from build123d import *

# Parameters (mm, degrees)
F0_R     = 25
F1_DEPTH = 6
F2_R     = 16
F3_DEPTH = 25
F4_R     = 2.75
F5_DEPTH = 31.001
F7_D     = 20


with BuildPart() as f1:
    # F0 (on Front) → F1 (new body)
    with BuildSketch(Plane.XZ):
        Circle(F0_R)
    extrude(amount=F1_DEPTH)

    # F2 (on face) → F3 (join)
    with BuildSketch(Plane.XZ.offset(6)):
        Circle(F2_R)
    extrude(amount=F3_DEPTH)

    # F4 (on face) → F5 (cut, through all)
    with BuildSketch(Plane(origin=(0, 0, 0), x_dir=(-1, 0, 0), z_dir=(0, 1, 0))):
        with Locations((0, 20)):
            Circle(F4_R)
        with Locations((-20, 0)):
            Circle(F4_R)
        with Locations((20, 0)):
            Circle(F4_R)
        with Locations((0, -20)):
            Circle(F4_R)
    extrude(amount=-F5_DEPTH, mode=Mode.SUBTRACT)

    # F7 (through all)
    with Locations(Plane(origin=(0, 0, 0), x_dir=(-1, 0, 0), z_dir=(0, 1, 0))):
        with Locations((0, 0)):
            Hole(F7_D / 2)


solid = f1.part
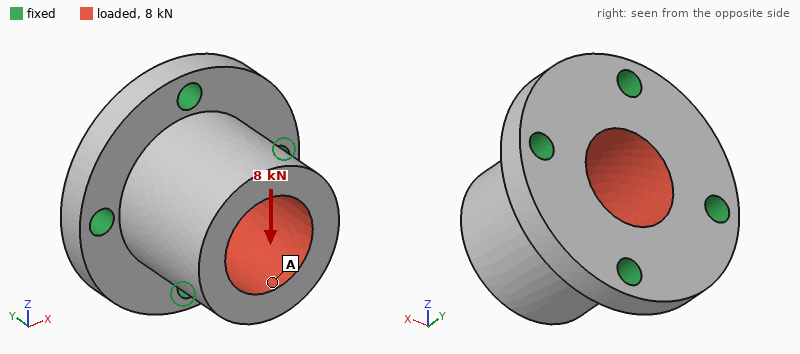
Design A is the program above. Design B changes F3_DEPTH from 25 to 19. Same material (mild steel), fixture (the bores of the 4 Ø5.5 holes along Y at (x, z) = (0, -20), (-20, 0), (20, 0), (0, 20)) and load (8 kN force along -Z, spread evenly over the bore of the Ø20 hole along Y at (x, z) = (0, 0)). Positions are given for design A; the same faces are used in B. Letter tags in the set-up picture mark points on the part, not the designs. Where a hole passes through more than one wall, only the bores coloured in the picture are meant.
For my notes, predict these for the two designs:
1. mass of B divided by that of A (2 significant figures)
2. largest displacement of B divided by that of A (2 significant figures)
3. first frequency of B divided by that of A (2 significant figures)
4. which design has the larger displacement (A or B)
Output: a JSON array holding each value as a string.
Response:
["0.86", "0.67", "1.3", "A"]
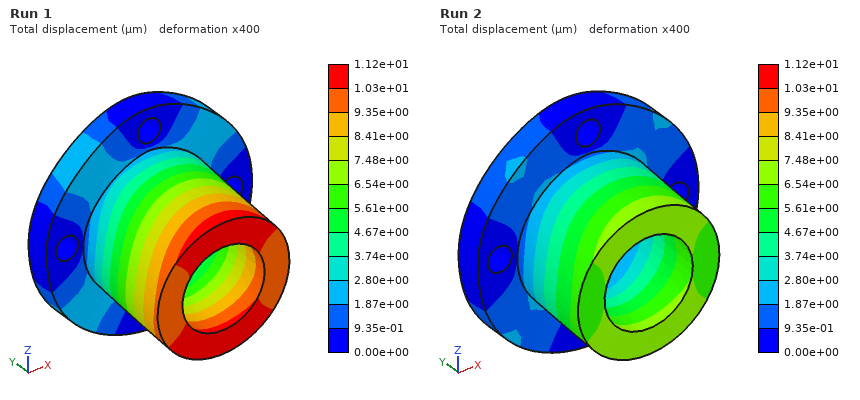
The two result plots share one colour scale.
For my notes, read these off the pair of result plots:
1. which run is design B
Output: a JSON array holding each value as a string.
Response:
["Run 2"]
